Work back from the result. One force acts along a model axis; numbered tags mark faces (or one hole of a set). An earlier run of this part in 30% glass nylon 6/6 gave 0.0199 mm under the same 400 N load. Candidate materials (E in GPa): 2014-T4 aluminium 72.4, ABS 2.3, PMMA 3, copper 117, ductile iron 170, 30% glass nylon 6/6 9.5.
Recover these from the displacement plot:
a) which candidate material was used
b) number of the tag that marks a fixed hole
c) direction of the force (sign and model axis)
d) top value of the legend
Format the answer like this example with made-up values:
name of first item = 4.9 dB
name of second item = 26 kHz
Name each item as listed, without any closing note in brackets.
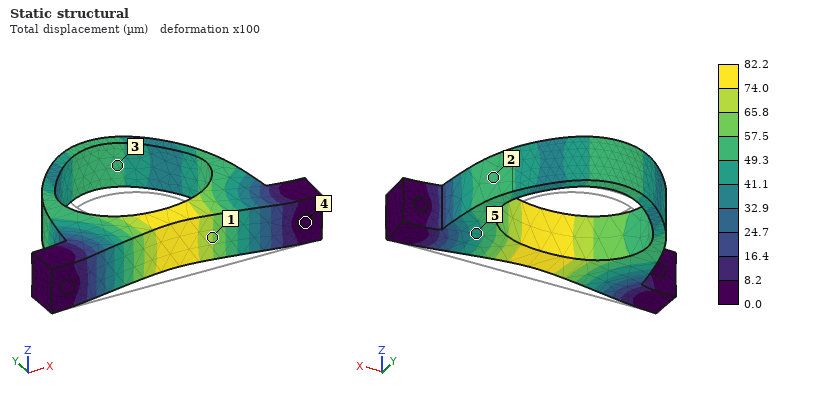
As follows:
which candidate material was used = ABS
number of the tag that marks a fixed hole = 4
direction of the force = +Y
top value of the legend = 82.2 µm
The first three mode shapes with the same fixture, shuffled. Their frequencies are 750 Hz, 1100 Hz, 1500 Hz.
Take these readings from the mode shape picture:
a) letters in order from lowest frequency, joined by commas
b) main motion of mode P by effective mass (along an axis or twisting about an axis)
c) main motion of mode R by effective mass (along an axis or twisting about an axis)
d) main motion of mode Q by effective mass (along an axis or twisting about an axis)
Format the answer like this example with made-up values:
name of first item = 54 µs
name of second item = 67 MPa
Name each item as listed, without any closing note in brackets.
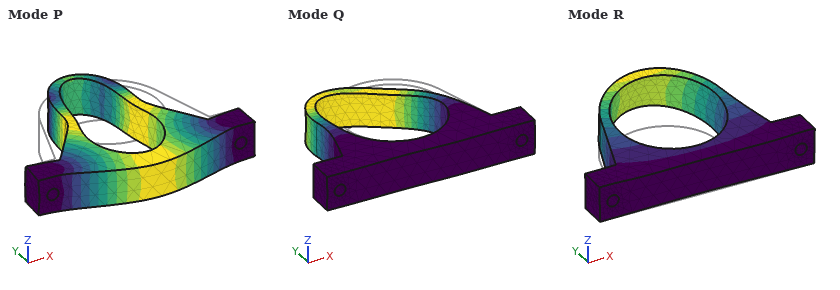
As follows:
letters in order from lowest frequency, joined by commas = R, Q, P
main motion of mode P by effective mass = along Y
main motion of mode R by effective mass = along Z
main motion of mode Q by effective mass = along X
